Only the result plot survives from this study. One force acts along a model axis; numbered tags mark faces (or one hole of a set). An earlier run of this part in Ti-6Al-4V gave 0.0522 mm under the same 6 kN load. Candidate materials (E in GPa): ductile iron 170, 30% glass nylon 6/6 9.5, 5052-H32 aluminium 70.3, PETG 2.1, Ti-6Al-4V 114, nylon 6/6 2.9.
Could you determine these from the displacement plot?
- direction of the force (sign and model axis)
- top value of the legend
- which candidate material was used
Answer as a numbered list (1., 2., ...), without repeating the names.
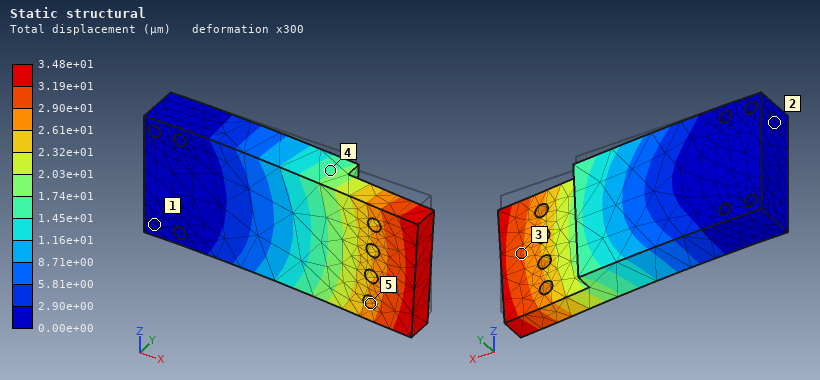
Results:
1. -Z
2. 3.48e+01 µm
3. ductile iron
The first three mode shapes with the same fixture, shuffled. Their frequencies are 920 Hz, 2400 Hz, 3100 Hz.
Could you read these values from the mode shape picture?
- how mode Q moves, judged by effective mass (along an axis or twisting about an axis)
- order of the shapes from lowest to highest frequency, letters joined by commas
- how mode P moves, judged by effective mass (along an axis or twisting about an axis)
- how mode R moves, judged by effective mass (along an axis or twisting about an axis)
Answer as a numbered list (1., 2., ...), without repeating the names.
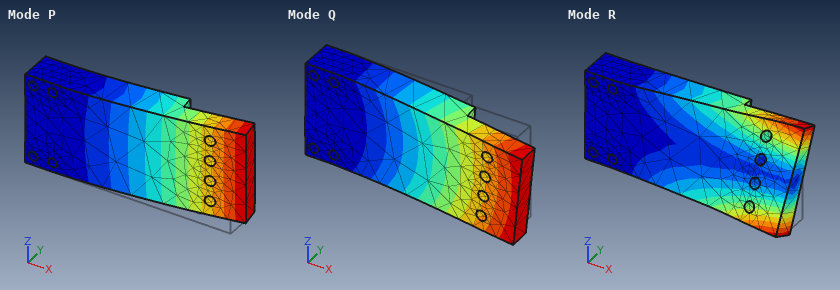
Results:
1. along Z
2. P, Q, R
3. along Y
4. twisting about X
